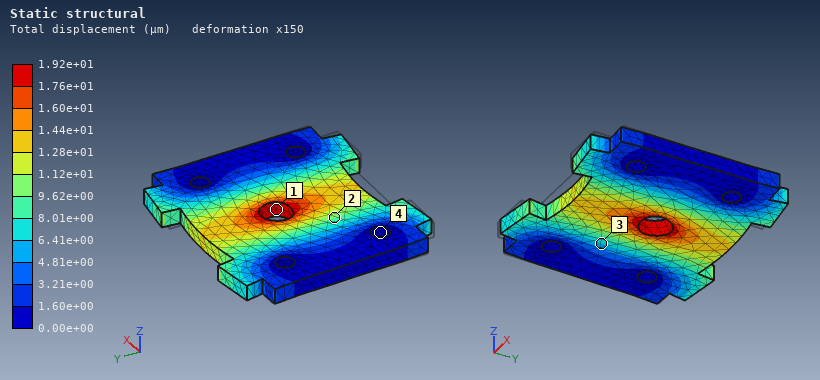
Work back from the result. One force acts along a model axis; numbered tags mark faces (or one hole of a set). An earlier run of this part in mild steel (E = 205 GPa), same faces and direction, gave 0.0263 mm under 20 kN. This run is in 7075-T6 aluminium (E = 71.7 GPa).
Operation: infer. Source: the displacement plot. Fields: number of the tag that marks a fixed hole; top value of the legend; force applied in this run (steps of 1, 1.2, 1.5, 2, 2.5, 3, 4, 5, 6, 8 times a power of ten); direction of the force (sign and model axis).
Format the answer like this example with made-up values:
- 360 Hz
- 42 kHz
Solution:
- 4
- 1.92e+01 µm
- 5 kN
- +Y
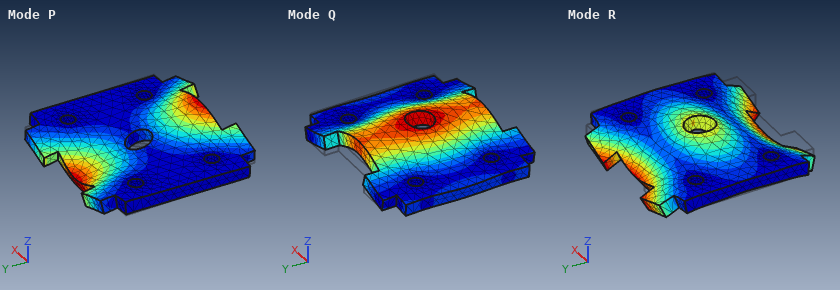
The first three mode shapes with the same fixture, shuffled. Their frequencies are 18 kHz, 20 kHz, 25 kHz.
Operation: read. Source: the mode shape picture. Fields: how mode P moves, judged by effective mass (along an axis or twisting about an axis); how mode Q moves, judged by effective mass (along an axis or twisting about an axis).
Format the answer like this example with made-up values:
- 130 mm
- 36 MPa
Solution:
- twisting about X
- along Z
